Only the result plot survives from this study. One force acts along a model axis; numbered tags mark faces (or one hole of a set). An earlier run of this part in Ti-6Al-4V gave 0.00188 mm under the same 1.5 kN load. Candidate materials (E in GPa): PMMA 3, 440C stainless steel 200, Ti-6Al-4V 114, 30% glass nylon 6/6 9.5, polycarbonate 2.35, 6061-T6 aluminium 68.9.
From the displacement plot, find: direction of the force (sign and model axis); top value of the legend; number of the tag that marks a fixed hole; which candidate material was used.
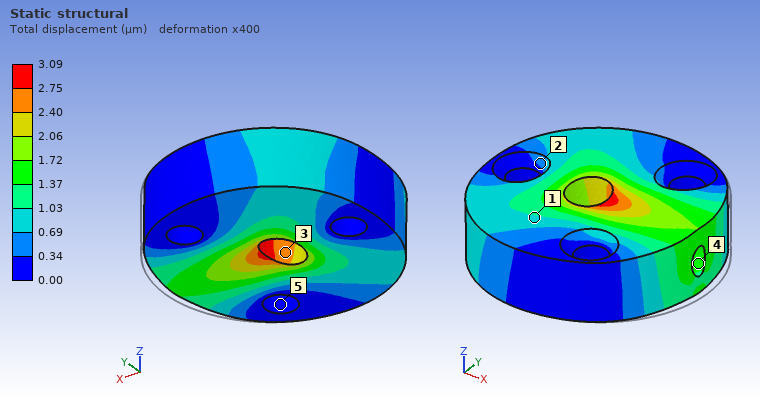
-X
3.09 µm
5
6061-T6 aluminium
